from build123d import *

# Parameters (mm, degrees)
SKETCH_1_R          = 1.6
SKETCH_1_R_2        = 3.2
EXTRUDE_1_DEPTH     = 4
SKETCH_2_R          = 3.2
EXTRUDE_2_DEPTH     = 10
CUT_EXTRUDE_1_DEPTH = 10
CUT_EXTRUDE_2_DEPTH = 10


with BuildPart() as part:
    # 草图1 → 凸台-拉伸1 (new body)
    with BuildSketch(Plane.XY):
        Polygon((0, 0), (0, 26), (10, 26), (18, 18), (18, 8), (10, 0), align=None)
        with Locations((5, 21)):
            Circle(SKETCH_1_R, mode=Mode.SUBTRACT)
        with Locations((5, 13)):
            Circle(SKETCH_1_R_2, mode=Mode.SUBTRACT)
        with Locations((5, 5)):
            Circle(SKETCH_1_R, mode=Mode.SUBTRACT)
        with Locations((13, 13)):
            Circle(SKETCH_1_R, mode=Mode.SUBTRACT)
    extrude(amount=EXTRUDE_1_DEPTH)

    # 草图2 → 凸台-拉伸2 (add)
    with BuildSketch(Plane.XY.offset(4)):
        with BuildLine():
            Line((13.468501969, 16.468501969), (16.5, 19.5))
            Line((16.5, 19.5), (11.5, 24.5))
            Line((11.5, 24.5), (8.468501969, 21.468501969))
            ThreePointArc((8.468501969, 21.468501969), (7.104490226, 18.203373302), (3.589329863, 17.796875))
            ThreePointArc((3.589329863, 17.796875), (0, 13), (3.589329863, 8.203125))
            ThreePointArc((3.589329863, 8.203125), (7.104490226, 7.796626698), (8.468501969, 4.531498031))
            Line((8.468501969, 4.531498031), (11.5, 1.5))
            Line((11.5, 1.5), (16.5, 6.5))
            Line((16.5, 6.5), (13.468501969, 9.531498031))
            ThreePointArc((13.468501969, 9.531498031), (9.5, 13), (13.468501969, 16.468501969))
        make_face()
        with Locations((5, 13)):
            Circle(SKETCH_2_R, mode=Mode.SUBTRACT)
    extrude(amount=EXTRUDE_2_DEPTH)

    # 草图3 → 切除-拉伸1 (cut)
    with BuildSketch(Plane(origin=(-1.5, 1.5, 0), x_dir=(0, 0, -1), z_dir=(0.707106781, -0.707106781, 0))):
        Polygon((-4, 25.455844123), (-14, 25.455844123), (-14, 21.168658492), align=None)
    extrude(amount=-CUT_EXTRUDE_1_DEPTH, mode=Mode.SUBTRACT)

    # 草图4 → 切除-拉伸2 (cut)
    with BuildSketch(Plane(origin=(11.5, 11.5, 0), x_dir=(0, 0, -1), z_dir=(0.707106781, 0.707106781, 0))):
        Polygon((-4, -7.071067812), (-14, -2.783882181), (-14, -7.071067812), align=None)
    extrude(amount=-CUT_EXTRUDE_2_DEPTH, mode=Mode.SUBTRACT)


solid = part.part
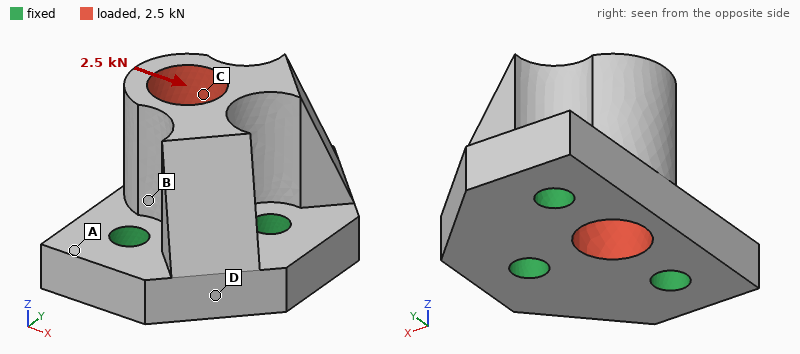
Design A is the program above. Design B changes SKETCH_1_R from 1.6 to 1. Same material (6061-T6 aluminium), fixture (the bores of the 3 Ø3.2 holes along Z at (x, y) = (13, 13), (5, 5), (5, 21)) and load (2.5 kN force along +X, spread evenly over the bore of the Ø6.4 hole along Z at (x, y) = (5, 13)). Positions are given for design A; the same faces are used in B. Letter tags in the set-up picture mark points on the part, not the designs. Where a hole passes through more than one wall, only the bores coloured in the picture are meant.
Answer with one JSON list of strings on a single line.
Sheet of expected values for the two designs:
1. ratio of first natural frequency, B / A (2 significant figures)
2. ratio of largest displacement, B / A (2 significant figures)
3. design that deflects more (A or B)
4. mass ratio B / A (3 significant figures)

["0.88", "1.2", "B", "1.02"]
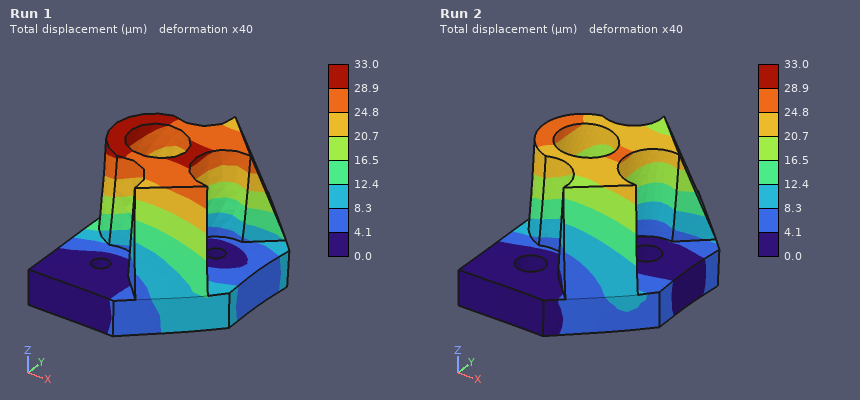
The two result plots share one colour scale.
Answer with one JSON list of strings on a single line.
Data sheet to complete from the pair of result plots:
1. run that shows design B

["Run 1"]
